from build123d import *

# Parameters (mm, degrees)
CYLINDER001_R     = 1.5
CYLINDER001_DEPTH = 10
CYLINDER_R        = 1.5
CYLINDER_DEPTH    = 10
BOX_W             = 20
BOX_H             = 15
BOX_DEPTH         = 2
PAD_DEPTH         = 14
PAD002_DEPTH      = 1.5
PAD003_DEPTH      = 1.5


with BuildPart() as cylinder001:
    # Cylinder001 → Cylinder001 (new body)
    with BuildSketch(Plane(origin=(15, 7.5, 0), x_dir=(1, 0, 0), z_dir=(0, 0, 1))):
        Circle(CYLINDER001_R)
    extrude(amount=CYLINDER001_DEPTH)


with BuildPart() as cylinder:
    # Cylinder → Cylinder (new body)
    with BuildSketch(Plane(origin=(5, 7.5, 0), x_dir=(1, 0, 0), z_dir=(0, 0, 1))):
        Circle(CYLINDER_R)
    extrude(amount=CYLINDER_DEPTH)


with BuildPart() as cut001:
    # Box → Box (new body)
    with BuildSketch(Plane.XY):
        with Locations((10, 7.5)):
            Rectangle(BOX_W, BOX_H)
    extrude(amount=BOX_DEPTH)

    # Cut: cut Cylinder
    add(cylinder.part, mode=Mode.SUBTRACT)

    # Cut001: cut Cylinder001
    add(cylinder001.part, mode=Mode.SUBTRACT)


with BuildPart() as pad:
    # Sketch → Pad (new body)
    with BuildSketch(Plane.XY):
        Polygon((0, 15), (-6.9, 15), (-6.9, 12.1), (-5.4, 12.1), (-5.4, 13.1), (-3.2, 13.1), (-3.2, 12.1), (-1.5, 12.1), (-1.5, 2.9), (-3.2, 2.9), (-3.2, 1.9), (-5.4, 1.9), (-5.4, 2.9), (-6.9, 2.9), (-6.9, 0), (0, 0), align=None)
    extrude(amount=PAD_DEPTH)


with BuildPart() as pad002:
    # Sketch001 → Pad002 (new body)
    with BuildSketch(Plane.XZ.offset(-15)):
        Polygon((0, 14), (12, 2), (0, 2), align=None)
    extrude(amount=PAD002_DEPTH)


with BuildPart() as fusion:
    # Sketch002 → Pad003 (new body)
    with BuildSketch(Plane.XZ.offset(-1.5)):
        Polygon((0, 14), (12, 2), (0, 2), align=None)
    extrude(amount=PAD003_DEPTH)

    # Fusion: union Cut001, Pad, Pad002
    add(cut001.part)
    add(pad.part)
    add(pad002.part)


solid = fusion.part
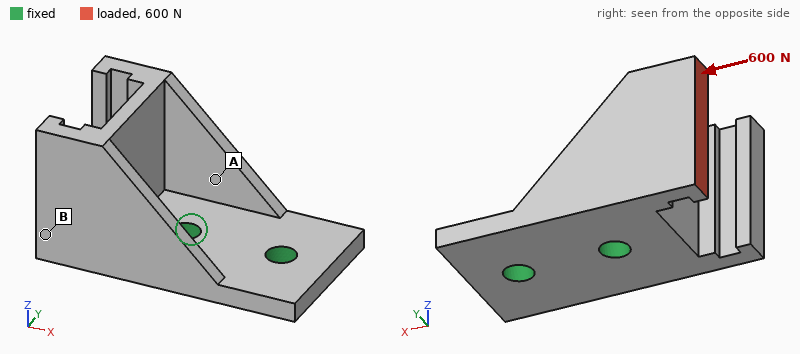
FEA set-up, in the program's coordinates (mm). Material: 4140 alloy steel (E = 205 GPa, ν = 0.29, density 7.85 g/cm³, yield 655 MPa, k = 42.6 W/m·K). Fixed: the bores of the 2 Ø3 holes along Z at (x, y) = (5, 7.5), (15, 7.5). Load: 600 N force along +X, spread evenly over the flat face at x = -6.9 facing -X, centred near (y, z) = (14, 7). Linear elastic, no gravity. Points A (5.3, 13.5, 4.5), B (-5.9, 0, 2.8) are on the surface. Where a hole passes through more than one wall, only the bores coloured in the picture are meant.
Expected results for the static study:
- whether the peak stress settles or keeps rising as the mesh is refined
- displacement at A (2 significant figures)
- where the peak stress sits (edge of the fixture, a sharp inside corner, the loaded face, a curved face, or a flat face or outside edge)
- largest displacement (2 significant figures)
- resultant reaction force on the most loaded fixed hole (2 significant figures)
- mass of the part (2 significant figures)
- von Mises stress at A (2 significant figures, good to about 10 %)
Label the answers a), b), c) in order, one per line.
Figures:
a) keeps rising
b) 11 µm
c) edge of the fixture
d) 53 µm
e) 500 N
f) 12 g
g) 72 MPa
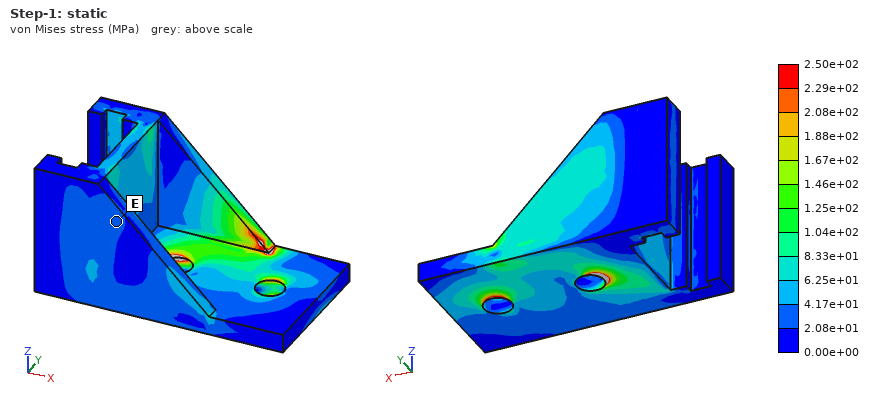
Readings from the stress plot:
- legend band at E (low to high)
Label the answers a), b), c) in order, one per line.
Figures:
a) 2.08e+01 to 4.17e+01 MPa
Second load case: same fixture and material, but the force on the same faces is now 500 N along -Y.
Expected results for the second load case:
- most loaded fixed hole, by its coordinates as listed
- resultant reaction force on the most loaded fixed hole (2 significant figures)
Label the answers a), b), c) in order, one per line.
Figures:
a) (5, 7.5)
b) 910 N
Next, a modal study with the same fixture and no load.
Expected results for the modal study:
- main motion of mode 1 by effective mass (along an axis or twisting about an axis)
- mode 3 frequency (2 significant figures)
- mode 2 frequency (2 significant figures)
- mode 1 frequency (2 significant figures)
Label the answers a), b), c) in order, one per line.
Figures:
a) along Y
b) 17 kHz
c) 8700 Hz
d) 6400 Hz
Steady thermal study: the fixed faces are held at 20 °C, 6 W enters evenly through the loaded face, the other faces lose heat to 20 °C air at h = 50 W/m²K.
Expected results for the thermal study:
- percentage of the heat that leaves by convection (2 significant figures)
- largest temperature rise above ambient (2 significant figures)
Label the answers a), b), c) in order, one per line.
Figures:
a) 25 %
b) 64 K
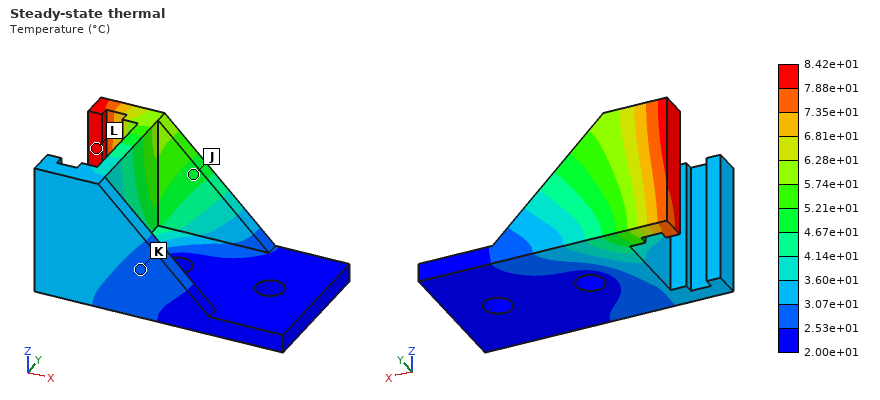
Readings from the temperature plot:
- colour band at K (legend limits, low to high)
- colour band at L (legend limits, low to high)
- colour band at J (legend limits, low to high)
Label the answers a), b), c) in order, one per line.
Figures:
a) 2.53e+01 to 3.07e+01 °C
b) 7.88e+01 to 8.42e+01 °C
c) 4.67e+01 to 5.21e+01 °C
